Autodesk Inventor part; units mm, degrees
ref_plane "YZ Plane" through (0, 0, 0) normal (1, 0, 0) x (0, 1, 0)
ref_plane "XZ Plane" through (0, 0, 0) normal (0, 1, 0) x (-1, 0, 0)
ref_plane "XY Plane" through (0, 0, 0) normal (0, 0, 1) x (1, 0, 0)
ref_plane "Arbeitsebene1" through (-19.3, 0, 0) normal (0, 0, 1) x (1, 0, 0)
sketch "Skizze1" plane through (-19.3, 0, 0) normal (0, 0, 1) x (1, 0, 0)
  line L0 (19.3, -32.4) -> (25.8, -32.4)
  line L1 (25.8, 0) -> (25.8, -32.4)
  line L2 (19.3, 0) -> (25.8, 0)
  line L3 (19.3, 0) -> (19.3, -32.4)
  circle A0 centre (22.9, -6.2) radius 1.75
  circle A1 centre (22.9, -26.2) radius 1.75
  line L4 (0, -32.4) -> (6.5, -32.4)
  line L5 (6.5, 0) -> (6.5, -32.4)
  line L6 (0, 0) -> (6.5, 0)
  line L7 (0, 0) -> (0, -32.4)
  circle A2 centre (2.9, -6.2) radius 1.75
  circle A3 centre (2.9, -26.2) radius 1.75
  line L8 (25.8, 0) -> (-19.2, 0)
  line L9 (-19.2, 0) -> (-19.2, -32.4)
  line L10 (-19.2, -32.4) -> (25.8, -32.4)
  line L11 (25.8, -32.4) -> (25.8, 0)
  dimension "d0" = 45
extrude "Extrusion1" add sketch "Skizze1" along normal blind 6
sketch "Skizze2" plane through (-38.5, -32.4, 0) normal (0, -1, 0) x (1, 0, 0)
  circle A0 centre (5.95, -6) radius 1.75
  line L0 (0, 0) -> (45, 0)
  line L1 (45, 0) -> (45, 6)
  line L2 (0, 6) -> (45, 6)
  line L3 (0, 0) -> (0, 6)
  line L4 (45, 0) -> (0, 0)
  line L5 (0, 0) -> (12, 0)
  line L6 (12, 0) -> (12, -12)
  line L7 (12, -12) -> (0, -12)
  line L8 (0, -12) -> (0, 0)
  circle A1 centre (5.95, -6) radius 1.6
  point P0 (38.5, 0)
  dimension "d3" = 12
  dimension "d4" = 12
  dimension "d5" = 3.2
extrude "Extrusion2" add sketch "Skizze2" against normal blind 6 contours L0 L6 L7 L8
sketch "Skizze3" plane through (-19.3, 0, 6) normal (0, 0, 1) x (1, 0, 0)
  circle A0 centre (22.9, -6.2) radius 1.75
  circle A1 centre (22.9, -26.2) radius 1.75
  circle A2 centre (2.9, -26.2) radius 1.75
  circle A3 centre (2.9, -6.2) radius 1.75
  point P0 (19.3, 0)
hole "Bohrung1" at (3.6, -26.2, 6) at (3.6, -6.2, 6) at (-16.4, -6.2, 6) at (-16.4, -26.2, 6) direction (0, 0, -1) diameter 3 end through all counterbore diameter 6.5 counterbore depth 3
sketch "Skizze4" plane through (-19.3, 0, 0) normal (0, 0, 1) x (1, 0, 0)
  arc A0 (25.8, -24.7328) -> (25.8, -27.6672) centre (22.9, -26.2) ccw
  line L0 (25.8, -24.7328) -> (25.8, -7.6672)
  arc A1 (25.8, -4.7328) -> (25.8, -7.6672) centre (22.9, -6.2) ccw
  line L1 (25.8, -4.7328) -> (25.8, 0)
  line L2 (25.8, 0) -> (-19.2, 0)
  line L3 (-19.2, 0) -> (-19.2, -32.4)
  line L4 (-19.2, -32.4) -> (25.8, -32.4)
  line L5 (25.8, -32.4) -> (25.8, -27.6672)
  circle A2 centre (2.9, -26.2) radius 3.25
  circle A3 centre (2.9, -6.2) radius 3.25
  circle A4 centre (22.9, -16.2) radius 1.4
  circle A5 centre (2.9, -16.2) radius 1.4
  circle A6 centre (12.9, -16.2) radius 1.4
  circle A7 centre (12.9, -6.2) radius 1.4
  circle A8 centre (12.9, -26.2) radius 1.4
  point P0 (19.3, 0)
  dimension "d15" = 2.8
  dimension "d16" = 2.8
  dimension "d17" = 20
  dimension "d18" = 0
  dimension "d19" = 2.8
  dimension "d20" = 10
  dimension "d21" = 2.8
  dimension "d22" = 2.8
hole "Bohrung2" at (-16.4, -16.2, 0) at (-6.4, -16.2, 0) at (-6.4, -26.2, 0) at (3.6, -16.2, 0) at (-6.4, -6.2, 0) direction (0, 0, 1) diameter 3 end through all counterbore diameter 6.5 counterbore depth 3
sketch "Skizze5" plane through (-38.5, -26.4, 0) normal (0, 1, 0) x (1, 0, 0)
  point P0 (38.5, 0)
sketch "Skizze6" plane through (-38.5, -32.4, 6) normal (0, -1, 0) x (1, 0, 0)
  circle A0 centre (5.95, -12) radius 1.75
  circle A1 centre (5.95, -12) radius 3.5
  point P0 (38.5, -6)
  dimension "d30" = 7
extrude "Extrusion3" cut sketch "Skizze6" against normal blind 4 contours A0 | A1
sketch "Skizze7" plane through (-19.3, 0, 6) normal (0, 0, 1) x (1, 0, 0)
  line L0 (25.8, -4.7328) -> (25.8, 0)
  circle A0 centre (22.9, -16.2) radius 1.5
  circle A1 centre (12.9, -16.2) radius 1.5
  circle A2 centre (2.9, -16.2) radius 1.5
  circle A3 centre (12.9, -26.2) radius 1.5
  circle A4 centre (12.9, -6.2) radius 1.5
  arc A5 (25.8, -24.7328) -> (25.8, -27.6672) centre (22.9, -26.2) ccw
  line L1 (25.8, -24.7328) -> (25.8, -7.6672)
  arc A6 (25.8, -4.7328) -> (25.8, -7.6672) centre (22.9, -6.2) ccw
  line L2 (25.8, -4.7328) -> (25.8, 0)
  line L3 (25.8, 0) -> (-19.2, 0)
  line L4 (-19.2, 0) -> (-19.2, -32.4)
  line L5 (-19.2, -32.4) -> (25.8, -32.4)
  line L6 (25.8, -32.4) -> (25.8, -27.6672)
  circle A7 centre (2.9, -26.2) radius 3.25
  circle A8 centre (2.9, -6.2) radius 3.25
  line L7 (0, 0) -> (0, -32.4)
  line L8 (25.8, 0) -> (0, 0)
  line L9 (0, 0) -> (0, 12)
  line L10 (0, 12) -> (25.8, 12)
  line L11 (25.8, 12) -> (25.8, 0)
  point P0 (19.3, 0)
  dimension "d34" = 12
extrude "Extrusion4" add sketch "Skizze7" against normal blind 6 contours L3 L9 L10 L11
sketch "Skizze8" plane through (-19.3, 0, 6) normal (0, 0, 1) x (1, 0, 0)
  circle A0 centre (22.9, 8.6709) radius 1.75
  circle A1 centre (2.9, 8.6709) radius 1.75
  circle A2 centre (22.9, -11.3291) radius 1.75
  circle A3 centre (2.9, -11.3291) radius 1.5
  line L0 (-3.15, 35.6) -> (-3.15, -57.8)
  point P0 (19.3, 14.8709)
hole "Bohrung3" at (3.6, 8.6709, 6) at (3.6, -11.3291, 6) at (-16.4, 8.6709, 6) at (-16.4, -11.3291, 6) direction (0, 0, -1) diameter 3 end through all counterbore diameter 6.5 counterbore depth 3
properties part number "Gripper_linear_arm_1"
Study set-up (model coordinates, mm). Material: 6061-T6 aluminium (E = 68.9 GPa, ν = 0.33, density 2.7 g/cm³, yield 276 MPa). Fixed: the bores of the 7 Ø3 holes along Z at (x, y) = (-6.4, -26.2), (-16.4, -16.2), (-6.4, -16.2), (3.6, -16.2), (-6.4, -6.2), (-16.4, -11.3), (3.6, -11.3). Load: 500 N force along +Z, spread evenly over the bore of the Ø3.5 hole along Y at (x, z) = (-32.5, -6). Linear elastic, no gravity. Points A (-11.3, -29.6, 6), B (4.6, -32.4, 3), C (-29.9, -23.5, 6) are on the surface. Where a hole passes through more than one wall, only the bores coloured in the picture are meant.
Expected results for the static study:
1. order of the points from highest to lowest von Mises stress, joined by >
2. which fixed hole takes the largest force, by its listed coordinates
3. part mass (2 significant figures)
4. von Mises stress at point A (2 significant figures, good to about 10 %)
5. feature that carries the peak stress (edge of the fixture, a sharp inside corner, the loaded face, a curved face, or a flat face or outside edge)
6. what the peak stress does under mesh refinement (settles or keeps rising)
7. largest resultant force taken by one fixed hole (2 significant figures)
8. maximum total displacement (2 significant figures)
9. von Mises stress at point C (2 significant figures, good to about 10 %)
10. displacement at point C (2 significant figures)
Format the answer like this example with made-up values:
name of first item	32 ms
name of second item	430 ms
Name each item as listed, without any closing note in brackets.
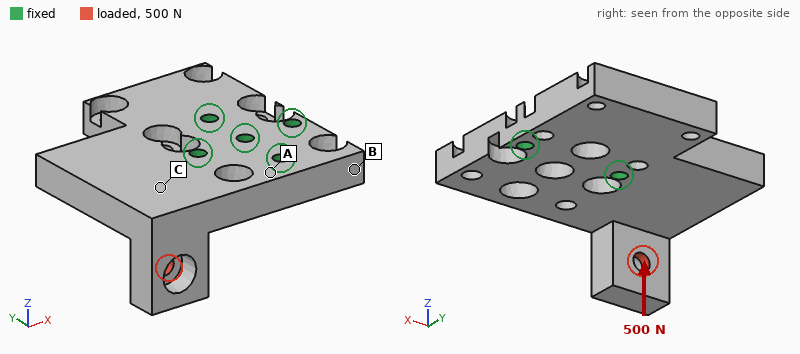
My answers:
order of the points from highest to lowest von Mises stress, joined by >	A > C > B
which fixed hole takes the largest force, by its listed coordinates	(-16.4, -16.2)
part mass	26 g
von Mises stress at point A	39 MPa
feature that carries the peak stress	edge of the fixture
what the peak stress does under mesh refinement	keeps rising
largest resultant force taken by one fixed hole	1.2 kN
maximum total displacement	0.12 mm
von Mises stress at point C	21 MPa
displacement at point C	0.051 mm
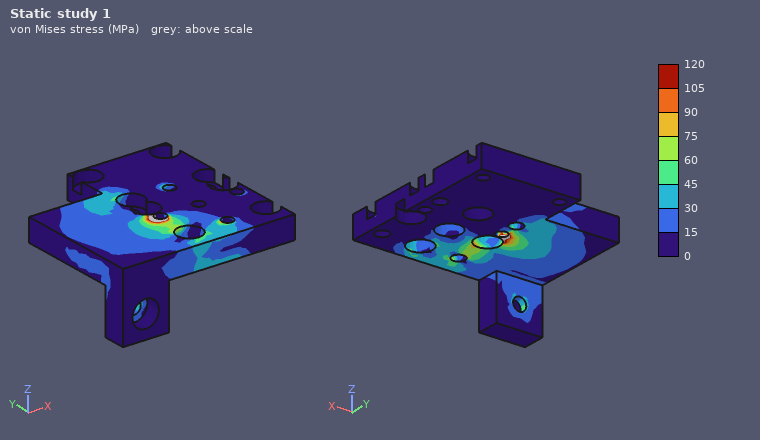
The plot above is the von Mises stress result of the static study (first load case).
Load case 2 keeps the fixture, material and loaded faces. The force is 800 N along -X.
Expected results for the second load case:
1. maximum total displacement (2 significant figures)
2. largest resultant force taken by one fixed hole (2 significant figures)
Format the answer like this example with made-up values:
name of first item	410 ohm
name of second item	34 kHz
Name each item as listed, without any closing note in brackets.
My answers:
maximum total displacement	0.13 mm
largest resultant force taken by one fixed hole	640 N
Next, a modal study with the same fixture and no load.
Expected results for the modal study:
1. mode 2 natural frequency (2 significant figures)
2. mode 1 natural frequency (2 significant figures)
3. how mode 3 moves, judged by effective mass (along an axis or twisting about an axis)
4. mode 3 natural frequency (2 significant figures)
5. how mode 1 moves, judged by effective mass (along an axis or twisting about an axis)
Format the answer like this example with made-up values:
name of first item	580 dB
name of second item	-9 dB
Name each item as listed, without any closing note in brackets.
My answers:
mode 2 natural frequency	8400 Hz
mode 1 natural frequency	5100 Hz
how mode 3 moves, judged by effective mass	along Z
mode 3 natural frequency	10 kHz
how mode 1 moves, judged by effective mass	along Z
